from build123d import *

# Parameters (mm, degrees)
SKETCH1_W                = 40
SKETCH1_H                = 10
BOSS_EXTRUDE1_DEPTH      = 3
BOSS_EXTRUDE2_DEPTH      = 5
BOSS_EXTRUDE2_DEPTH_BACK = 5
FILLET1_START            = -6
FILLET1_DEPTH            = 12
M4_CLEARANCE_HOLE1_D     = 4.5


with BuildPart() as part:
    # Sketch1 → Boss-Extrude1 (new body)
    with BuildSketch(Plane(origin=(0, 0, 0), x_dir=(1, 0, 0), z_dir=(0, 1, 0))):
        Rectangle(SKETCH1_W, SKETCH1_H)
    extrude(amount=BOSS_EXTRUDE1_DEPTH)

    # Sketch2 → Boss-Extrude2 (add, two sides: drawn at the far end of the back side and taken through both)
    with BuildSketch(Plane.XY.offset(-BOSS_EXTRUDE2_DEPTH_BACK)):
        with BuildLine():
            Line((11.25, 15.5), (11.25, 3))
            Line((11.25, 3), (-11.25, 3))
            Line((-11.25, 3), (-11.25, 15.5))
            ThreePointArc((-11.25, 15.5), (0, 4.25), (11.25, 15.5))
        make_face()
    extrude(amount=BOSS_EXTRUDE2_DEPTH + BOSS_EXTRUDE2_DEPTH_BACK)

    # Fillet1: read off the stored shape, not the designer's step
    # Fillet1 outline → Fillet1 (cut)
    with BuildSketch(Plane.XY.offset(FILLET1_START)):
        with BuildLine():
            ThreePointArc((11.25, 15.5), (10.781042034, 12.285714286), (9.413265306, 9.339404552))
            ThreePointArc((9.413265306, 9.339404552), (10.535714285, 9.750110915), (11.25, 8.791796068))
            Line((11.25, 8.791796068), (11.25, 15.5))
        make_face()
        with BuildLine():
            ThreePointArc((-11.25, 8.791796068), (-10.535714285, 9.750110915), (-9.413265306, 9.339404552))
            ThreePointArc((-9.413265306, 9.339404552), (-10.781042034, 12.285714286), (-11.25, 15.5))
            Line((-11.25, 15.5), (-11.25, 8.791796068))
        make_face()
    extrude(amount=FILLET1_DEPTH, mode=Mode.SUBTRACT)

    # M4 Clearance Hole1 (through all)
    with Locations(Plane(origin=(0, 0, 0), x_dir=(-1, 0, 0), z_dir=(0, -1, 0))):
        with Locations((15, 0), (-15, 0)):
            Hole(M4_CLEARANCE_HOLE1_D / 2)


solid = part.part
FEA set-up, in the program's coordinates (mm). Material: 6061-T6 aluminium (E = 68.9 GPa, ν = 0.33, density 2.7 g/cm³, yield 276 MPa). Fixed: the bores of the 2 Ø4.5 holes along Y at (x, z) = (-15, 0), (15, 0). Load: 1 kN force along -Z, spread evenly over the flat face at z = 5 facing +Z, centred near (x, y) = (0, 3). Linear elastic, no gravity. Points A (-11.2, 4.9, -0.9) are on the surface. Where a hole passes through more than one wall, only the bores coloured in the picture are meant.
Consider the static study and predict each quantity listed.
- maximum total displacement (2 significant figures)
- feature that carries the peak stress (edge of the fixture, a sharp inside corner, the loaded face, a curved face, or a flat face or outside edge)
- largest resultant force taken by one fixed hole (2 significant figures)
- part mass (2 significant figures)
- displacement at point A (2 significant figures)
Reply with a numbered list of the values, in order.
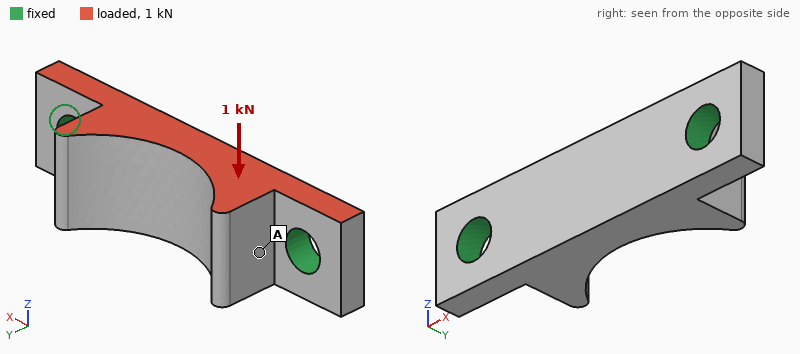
1. 11 µm
2. edge of the fixture
3. 500 N
4. 5.0 g
5. 5.5 µm
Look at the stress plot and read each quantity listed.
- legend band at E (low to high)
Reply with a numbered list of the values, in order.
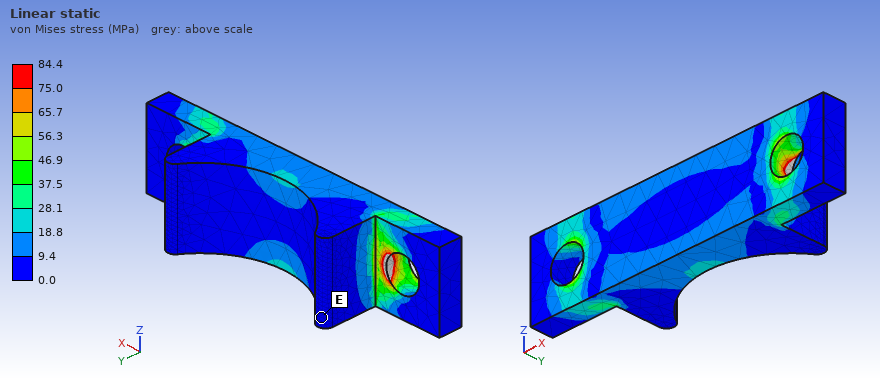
1. 0.0 to 9.4 MPa
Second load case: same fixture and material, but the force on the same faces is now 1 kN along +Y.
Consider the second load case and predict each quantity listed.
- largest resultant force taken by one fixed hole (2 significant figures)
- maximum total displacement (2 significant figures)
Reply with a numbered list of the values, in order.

1. 550 N
2. 31 µm
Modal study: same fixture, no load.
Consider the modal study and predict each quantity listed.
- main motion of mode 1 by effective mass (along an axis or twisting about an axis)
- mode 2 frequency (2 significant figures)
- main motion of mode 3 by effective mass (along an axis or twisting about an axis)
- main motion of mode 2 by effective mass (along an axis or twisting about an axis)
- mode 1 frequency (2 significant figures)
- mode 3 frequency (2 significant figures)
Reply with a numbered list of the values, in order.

1. along Y
2. 23 kHz
3. along Z
4. along Z
5. 20 kHz
6. 34 kHz
